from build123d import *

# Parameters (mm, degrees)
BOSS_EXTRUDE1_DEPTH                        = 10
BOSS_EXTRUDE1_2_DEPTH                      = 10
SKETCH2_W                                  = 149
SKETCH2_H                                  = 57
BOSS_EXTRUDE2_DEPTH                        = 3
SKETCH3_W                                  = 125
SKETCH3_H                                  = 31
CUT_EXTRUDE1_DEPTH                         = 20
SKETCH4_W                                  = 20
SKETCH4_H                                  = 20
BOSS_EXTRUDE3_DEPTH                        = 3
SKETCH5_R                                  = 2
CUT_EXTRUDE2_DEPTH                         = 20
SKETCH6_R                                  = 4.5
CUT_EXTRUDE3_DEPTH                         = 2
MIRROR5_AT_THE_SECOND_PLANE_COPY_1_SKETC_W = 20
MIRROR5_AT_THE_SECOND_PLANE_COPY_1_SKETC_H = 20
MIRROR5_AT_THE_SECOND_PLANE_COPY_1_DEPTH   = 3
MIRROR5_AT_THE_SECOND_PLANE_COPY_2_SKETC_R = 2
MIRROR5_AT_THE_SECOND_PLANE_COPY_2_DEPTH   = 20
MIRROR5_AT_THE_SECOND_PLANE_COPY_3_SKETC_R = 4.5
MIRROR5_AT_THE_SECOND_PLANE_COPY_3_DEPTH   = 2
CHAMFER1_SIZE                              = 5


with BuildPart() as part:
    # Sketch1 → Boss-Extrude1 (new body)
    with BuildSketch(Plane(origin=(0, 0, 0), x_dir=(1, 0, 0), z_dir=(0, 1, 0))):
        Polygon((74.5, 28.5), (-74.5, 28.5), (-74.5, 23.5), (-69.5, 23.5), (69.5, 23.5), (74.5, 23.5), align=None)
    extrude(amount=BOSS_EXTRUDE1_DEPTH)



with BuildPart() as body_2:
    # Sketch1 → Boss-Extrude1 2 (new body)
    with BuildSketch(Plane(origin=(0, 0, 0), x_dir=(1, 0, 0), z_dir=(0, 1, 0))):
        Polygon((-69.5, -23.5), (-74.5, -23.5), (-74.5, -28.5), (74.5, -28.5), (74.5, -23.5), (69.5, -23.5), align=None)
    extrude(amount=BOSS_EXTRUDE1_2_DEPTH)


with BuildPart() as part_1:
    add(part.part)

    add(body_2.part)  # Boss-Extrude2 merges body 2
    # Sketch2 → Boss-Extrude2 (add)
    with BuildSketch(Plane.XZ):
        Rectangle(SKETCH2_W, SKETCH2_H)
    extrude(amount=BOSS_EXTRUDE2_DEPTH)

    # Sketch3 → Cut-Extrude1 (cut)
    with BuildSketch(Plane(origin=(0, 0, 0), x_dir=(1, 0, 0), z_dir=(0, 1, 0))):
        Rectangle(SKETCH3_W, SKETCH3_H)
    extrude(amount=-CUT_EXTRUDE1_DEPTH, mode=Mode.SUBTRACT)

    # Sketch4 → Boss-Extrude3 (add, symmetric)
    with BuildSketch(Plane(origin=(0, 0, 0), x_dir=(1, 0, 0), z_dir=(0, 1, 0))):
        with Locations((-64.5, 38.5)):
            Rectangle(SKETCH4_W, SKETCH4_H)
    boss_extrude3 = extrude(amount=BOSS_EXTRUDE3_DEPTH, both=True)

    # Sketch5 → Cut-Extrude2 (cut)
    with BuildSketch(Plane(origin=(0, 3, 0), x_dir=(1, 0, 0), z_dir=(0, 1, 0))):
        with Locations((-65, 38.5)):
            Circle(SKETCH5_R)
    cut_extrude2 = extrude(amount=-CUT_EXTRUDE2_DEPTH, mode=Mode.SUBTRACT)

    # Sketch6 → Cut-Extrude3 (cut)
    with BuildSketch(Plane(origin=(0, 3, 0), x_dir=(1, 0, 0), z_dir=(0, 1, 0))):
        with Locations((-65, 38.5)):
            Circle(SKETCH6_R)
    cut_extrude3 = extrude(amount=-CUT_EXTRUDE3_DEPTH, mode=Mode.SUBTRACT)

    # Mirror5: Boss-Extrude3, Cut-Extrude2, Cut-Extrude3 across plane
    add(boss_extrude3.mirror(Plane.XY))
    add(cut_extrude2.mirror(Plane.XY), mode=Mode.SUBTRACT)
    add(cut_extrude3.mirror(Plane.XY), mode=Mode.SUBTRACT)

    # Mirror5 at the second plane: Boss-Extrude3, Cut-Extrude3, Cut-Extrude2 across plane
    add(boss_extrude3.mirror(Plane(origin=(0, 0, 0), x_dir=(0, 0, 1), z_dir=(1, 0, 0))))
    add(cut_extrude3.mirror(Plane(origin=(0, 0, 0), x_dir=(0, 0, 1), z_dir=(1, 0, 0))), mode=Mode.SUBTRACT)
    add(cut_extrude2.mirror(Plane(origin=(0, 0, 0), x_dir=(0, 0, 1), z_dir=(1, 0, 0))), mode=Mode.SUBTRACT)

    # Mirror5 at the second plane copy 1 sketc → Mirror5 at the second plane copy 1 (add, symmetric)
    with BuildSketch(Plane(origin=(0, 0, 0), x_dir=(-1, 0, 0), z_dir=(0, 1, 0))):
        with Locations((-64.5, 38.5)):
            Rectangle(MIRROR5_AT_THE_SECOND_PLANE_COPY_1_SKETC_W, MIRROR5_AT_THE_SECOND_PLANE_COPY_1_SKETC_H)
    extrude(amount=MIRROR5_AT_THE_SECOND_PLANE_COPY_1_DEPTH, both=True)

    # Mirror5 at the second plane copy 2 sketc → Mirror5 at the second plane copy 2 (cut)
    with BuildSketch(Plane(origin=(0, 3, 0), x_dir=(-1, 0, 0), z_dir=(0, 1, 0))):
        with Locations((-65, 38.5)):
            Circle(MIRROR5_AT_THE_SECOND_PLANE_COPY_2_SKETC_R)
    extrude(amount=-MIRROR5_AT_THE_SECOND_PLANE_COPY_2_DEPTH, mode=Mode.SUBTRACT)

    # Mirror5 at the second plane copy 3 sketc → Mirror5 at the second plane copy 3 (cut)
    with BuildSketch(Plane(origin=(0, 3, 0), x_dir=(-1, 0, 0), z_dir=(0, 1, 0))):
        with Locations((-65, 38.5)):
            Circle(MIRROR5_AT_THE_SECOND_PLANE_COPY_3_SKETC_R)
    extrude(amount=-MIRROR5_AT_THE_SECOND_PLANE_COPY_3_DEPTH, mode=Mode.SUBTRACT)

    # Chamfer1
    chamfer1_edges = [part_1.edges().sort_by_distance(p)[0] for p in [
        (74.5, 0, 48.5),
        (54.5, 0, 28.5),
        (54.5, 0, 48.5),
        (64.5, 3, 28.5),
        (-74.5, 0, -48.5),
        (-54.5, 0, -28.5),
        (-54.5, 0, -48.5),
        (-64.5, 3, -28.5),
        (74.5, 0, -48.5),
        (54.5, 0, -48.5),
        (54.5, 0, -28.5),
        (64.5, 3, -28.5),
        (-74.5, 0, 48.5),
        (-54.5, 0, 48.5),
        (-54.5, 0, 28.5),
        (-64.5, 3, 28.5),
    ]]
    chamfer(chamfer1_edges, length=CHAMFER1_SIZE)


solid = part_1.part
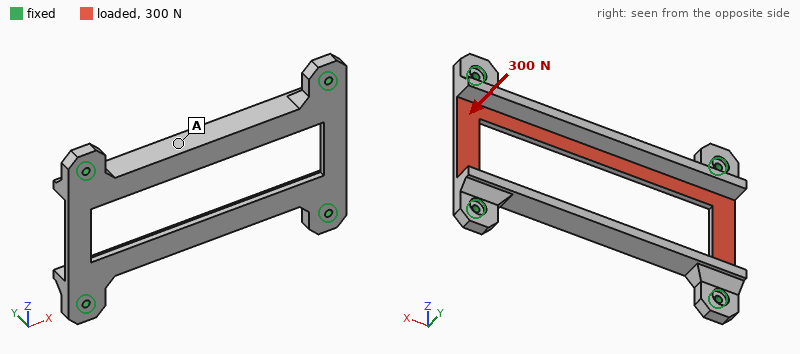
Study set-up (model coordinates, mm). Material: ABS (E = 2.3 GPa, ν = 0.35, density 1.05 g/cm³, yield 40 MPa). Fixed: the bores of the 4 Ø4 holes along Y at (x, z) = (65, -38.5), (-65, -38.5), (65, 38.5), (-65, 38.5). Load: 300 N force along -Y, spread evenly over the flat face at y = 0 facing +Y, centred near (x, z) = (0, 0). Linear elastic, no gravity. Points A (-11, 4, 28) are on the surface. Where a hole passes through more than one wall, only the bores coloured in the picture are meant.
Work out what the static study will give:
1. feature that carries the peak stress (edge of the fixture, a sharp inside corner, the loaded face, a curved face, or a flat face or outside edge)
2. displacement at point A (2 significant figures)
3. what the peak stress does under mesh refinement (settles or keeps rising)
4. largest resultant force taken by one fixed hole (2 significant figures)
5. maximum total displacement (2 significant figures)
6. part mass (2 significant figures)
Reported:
edge of the fixture
0.57 mm
keeps rising
94 N
1.1 mm
40 g
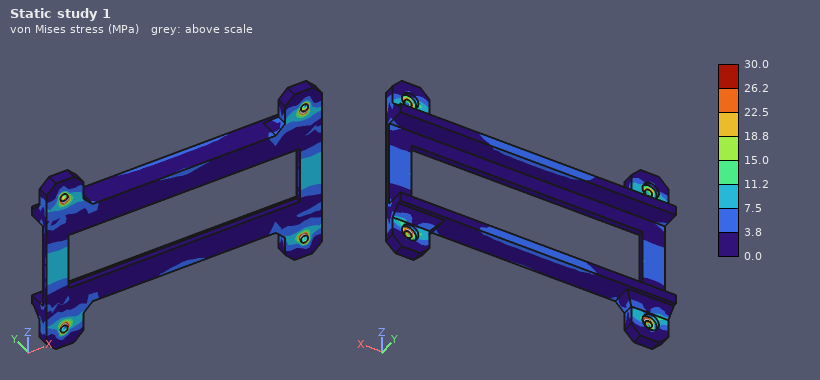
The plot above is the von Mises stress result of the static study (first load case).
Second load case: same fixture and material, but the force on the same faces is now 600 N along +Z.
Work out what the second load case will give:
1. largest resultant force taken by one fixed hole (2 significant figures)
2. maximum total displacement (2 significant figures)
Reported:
180 N
0.49 mm
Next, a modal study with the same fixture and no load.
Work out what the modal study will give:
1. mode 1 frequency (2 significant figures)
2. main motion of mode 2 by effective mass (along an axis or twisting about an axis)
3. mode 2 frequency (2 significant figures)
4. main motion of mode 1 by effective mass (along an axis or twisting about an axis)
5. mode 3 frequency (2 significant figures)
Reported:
650 Hz
twisting about X
680 Hz
along Y
980 Hz
